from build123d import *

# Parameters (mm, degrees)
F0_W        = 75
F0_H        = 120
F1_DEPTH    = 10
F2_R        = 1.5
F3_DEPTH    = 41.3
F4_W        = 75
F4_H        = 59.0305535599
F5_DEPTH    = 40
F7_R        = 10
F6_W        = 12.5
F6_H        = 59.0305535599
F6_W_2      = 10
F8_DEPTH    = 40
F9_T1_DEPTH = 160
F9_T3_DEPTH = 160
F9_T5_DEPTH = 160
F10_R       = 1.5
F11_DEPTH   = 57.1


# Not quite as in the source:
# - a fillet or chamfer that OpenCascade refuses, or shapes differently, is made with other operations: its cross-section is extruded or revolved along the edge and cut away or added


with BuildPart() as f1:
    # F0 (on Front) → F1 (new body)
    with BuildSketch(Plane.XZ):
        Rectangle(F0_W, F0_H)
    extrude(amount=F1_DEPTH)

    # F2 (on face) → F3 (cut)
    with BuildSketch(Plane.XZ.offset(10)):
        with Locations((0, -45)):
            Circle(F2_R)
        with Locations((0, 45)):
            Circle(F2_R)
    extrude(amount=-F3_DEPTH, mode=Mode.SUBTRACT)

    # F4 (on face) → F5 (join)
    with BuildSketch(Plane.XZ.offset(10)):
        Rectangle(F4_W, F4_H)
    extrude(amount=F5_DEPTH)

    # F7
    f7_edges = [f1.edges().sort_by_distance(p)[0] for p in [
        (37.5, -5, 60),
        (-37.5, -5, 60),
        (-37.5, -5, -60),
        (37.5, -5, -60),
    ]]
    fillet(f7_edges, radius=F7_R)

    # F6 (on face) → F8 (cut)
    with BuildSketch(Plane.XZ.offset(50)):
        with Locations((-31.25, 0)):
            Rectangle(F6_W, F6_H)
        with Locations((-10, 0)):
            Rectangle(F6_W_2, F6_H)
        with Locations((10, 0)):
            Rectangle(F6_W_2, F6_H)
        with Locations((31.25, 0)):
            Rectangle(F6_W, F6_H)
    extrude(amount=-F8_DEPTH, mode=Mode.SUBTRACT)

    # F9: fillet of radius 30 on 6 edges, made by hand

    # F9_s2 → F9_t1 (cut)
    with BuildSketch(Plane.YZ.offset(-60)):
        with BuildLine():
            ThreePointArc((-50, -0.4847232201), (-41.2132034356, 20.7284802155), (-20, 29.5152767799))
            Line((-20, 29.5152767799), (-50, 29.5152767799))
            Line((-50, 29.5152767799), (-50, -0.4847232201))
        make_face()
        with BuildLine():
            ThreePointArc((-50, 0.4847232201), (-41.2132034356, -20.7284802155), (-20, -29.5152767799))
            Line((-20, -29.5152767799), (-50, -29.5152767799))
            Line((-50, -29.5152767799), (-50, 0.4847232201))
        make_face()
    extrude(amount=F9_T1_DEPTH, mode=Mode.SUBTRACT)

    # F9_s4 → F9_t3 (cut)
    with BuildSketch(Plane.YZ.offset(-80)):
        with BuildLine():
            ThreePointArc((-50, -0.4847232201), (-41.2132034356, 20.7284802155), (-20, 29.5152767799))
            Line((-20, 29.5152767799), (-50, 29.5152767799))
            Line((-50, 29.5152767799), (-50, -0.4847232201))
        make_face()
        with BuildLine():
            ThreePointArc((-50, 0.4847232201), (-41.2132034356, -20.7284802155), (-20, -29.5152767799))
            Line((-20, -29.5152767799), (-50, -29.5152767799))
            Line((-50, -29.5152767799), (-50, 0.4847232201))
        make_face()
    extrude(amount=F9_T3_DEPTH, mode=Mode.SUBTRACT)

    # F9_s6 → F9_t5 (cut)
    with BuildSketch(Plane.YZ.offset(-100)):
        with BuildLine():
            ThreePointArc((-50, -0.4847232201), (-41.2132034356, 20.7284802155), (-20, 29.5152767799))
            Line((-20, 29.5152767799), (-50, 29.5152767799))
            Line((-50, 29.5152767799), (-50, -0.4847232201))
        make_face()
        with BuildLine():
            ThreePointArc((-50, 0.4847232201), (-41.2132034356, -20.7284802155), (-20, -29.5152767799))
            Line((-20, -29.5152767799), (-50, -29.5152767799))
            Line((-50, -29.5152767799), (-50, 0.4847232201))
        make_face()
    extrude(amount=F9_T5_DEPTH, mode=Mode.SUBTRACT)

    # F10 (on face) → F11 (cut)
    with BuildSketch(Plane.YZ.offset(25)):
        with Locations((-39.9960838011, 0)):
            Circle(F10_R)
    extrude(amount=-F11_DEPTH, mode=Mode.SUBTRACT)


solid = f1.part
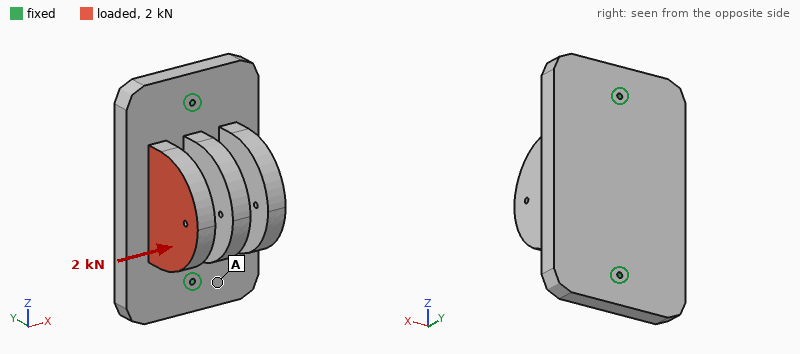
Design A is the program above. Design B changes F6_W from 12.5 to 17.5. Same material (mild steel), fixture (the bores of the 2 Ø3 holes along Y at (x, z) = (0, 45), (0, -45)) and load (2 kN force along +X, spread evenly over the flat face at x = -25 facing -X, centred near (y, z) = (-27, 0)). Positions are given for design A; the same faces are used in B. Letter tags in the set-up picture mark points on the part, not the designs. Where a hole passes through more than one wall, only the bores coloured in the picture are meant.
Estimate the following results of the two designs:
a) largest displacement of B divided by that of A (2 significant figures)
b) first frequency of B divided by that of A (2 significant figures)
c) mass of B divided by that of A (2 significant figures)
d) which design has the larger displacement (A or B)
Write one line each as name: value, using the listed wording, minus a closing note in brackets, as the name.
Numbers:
largest displacement of B divided by that of A: 1.3
first frequency of B divided by that of A: 1.1
mass of B divided by that of A: 0.93
which design has the larger displacement: B
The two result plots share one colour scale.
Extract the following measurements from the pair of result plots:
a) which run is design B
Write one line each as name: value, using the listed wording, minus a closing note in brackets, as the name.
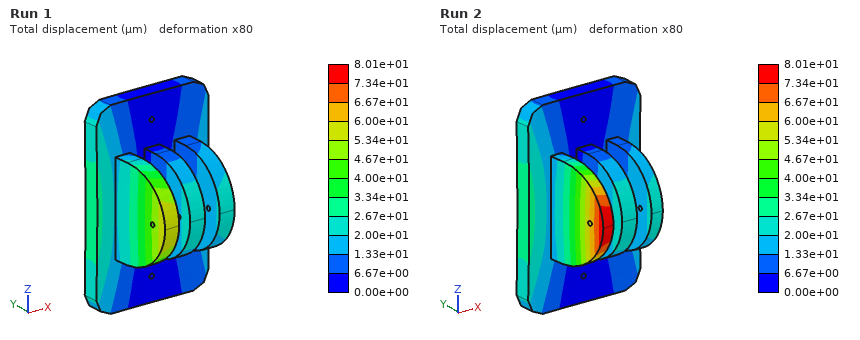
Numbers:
which run is design B: Run 2
